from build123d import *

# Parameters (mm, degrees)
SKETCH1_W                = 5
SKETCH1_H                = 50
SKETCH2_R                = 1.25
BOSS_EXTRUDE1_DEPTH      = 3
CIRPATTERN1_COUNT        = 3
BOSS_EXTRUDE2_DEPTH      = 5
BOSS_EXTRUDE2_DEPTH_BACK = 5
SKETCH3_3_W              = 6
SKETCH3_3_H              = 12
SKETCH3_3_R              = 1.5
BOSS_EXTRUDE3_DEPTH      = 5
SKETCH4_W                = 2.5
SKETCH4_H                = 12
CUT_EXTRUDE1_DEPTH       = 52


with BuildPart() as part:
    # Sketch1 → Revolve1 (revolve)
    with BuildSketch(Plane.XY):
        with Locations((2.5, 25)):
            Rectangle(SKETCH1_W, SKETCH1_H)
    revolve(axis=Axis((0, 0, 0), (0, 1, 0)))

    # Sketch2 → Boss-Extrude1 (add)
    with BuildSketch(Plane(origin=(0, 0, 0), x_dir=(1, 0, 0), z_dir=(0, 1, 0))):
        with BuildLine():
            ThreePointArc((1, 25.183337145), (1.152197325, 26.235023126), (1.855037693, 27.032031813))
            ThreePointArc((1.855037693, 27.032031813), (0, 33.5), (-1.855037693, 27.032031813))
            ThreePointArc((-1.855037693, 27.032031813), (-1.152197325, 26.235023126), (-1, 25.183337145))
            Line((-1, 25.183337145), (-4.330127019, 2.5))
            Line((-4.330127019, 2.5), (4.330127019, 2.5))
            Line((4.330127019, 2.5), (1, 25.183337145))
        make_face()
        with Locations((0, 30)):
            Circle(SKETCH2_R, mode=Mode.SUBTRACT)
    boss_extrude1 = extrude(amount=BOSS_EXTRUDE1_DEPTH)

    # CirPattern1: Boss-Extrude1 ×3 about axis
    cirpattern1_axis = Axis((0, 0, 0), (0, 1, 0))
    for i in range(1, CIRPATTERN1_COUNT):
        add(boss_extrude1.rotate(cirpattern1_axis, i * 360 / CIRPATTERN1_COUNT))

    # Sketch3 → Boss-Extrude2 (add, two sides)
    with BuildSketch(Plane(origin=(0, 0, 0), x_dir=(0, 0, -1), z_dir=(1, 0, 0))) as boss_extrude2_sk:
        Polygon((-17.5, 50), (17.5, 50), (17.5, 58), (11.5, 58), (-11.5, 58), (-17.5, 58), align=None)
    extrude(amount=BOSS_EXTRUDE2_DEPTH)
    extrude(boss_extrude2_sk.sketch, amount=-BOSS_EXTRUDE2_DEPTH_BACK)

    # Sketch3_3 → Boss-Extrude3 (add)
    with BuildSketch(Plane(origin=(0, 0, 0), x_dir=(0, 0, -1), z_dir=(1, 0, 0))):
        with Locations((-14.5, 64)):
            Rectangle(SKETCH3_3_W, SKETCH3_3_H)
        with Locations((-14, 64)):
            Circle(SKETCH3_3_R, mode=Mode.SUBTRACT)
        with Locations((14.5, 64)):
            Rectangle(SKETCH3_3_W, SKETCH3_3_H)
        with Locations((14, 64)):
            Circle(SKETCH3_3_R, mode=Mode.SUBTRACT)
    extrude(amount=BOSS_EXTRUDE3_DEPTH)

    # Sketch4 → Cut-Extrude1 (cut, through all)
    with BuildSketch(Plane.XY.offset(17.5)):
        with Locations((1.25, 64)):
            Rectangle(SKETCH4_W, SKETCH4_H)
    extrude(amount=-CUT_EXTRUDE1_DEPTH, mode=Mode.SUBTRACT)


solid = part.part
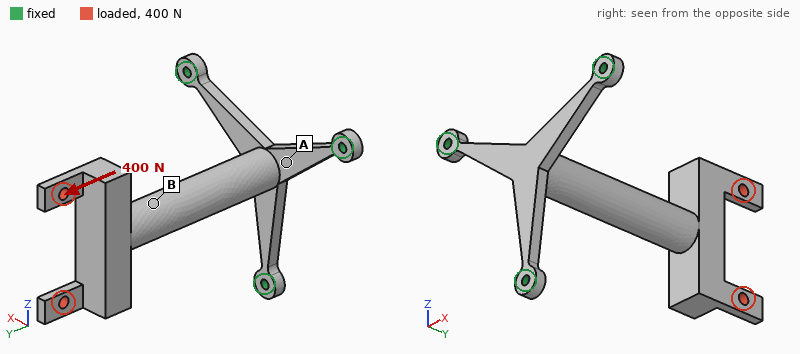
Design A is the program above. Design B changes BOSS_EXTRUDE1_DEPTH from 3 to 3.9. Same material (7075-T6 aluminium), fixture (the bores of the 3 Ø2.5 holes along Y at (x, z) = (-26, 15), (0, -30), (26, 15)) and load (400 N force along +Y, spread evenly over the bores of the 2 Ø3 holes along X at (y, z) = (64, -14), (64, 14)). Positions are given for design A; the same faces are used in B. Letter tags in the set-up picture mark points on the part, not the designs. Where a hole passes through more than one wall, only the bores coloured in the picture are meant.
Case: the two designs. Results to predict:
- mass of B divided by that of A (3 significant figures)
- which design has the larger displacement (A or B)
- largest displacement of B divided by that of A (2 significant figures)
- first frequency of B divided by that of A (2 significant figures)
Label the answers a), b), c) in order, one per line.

a) 1.05
b) A
c) 0.58
d) 1.3
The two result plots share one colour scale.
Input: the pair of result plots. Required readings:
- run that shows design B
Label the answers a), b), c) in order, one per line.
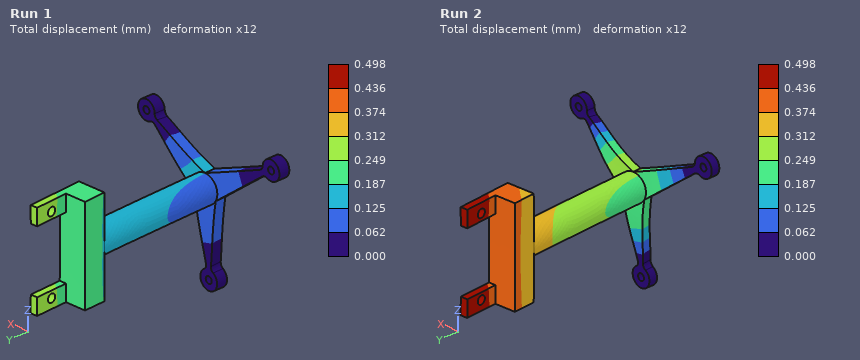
a) Run 1
